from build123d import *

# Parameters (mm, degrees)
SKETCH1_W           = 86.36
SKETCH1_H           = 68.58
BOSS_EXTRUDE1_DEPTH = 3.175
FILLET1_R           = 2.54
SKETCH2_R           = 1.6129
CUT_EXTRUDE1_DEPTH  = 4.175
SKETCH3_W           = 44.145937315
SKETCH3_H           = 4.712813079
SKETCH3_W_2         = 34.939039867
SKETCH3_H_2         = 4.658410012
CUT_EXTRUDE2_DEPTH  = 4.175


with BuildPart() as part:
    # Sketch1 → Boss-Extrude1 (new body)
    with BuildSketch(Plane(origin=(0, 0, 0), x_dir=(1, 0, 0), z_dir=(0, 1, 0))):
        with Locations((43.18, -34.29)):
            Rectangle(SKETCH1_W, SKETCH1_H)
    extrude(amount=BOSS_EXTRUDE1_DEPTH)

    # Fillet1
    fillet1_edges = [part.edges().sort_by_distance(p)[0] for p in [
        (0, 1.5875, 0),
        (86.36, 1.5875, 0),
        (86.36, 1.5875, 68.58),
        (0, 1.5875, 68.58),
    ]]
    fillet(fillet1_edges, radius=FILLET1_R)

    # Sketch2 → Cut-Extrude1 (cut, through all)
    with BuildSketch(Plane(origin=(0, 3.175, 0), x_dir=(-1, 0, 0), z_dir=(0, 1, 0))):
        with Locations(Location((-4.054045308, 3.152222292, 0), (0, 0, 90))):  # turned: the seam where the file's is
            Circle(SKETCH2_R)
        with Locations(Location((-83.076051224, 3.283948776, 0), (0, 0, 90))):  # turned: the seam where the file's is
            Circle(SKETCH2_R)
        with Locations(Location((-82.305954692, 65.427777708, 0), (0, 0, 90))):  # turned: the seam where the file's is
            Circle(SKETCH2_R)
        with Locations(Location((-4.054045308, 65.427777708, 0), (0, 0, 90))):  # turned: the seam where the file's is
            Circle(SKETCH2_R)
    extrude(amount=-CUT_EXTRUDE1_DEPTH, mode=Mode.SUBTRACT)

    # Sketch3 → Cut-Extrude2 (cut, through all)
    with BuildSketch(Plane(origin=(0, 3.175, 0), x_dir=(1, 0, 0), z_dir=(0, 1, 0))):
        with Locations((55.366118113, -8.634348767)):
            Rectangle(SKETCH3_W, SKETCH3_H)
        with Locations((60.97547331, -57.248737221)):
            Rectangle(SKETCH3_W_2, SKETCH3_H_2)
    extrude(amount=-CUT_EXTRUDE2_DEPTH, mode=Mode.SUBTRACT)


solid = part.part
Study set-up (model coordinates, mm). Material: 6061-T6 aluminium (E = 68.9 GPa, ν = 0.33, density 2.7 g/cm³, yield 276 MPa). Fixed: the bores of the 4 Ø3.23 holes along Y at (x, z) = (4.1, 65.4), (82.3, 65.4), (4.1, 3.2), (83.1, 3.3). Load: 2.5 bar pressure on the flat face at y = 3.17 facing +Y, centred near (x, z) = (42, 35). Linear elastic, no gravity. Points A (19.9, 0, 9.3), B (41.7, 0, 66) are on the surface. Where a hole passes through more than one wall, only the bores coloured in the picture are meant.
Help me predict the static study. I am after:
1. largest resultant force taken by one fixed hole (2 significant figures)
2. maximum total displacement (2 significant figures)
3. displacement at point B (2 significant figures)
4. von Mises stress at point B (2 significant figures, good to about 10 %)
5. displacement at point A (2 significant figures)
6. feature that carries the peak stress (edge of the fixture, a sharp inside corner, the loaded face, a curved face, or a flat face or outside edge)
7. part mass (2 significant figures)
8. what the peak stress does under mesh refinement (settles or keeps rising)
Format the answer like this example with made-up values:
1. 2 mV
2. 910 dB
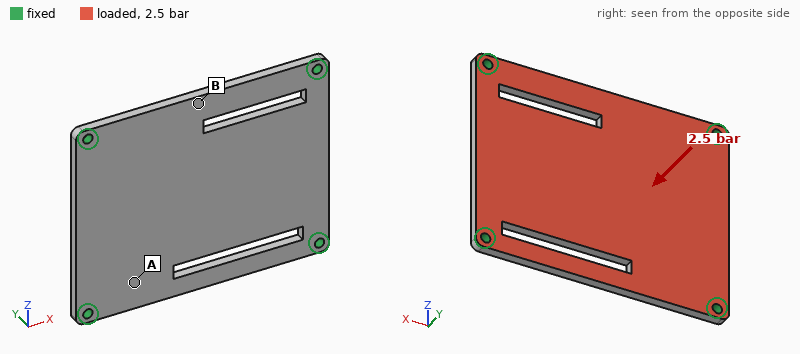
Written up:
1. 360 N
2. 0.30 mm
3. 0.22 mm
4. 69 MPa
5. 0.13 mm
6. edge of the fixture
7. 47 g
8. keeps rising
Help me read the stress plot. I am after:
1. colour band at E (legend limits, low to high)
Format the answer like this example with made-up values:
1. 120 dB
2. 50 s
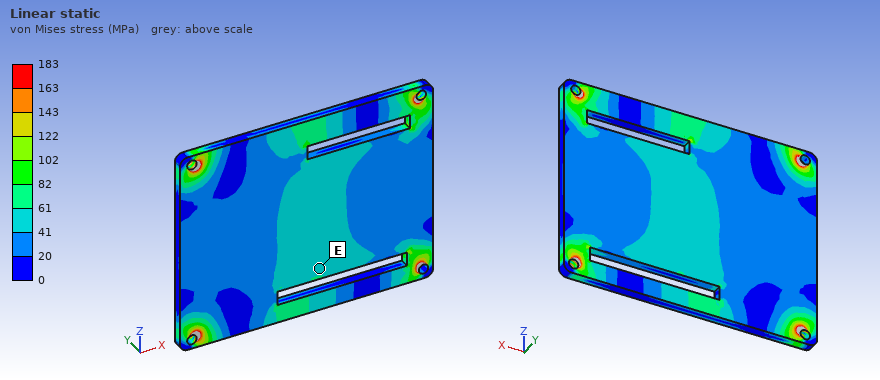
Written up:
1. 41 to 61 MPa
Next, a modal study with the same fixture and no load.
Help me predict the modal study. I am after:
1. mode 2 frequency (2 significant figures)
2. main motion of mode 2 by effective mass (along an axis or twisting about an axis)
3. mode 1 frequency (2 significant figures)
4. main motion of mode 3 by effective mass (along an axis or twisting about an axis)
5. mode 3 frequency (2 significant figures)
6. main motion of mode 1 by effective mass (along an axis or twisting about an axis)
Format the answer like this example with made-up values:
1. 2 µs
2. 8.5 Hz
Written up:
1. 3200 Hz
2. twisting about X
3. 1800 Hz
4. twisting about Z
5. 3800 Hz
6. along Y
